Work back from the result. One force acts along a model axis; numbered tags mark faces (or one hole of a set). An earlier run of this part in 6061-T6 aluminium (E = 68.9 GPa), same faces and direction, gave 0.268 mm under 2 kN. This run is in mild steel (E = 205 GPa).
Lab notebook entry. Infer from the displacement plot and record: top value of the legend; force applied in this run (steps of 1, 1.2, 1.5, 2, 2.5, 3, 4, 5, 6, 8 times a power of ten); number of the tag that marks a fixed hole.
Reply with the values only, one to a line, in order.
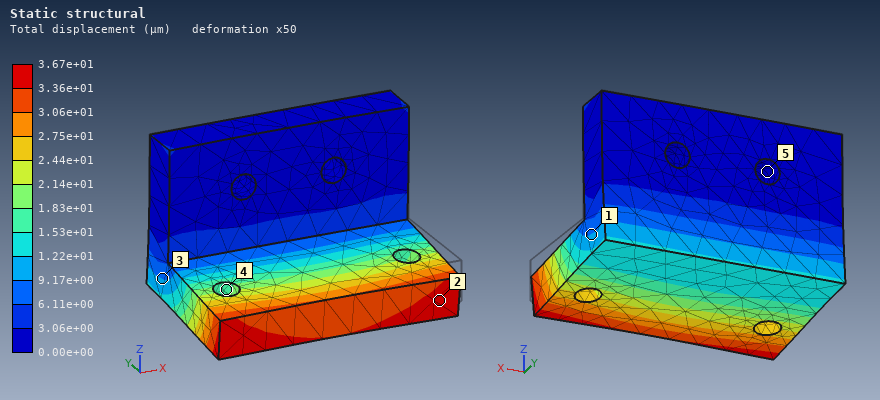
3.67e+01 µm
800 N
5
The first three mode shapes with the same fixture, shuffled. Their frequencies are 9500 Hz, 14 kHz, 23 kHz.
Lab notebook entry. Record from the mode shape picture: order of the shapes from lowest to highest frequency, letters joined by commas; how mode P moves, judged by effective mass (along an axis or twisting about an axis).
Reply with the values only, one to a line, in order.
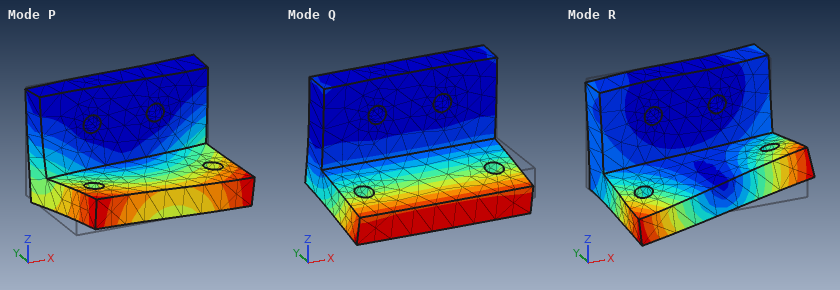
Q, P, R
along X
